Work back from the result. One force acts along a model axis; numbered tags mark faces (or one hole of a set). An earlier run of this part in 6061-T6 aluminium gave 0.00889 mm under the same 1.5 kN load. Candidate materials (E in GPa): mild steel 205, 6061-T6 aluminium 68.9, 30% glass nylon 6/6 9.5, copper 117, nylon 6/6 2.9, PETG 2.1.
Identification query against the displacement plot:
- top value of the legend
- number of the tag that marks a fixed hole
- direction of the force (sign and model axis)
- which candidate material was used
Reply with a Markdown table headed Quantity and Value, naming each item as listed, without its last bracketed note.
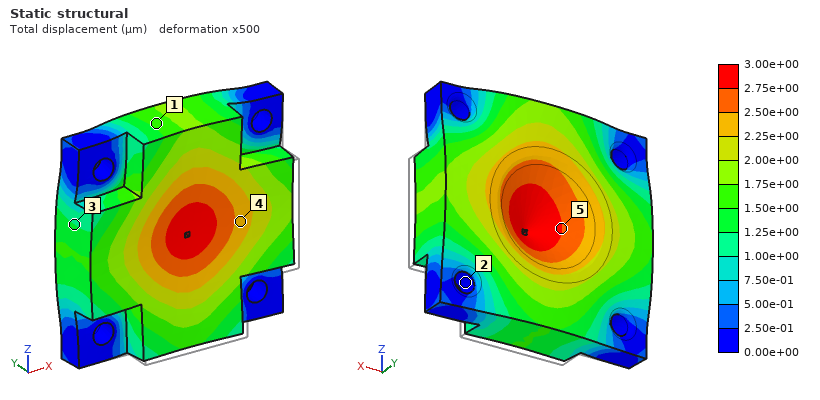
| Quantity | Value |
|---|---|
| top value of the legend | 3.00e+00 µm |
| number of the tag that marks a fixed hole | 2 |
| direction of the force | +Y |
| which candidate material was used | mild steel |
